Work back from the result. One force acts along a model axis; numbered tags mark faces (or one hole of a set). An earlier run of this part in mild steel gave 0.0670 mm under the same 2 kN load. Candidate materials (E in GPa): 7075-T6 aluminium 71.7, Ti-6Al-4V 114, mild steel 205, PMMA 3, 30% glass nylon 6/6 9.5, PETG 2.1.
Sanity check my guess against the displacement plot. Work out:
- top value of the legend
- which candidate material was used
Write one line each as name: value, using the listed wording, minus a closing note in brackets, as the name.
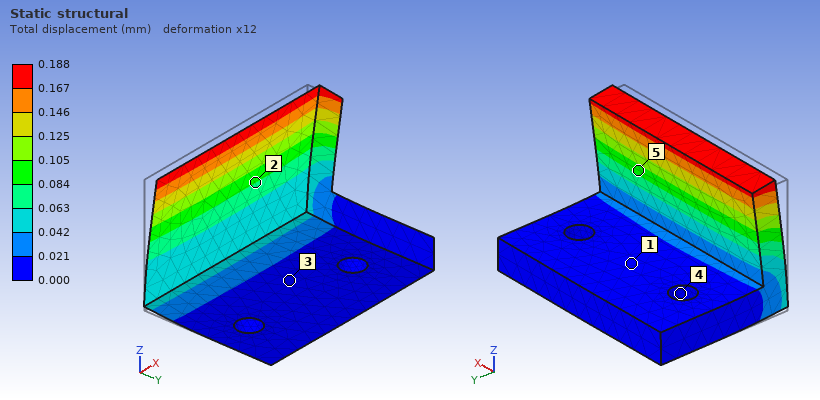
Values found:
top value of the legend: 0.188 mm
which candidate material was used: 7075-T6 aluminium
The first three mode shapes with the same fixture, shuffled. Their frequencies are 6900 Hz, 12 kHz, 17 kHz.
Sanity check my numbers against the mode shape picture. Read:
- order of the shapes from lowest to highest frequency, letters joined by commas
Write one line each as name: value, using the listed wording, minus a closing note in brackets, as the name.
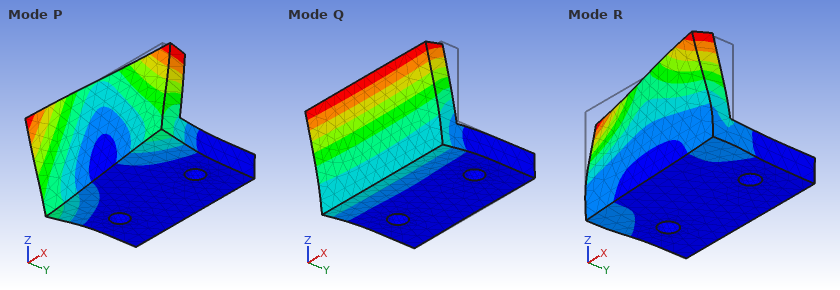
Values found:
order of the shapes from lowest to highest frequency, letters joined by commas: Q, P, R
